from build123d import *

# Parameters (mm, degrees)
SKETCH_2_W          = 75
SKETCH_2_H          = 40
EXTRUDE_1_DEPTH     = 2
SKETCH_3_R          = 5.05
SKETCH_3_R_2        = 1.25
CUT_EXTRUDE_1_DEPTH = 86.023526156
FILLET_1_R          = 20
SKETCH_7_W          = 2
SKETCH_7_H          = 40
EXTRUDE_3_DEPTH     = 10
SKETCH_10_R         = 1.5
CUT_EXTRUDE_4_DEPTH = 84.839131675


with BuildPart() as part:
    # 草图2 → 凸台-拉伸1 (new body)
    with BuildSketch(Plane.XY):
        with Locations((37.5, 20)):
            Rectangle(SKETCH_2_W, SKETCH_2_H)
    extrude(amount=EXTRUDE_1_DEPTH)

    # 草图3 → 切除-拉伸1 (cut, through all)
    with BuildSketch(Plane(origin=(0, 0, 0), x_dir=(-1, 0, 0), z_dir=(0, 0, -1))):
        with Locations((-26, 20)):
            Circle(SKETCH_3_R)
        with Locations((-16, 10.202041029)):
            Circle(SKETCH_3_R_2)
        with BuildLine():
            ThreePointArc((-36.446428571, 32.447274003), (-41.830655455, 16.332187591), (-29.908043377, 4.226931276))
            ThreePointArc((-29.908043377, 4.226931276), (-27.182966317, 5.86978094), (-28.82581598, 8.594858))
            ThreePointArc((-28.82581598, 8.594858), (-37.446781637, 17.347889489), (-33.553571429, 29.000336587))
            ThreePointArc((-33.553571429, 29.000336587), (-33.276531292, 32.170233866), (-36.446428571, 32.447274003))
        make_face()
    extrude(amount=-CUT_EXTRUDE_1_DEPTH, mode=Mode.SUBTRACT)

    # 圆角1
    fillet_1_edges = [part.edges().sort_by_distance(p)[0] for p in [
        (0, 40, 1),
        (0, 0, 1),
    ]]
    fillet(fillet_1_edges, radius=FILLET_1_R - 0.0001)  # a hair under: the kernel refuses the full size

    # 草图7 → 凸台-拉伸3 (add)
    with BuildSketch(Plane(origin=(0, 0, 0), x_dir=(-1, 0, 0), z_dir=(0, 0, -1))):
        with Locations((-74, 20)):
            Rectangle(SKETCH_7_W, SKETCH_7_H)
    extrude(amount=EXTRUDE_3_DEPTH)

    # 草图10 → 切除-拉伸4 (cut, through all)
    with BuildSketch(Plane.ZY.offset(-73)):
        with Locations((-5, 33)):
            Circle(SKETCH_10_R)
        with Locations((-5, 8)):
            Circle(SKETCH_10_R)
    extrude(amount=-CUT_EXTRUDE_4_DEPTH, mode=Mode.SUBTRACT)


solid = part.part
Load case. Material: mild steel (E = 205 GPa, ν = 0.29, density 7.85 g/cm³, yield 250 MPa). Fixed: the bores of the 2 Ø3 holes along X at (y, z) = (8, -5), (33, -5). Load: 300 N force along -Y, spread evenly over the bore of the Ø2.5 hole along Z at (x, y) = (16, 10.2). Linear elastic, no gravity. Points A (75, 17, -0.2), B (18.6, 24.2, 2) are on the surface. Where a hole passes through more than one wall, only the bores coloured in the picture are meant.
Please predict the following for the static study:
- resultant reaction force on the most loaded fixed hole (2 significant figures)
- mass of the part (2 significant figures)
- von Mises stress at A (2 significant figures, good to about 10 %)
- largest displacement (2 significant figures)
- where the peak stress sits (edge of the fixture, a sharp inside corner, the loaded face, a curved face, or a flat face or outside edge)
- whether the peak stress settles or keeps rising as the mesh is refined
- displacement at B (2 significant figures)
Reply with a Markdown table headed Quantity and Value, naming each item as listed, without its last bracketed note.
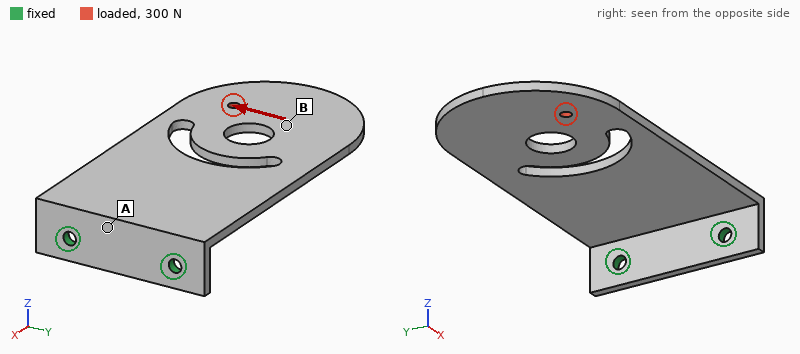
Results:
| Quantity | Value |
|---|---|
| resultant reaction force on the most loaded fixed hole | 670 N |
| mass of the part | 47 g |
| von Mises stress at A | 61 MPa |
| largest displacement | 0.12 mm |
| where the peak stress sits | edge of the fixture |
| whether the peak stress settles or keeps rising as the mesh is refined | keeps rising |
| displacement at B | 0.086 mm |
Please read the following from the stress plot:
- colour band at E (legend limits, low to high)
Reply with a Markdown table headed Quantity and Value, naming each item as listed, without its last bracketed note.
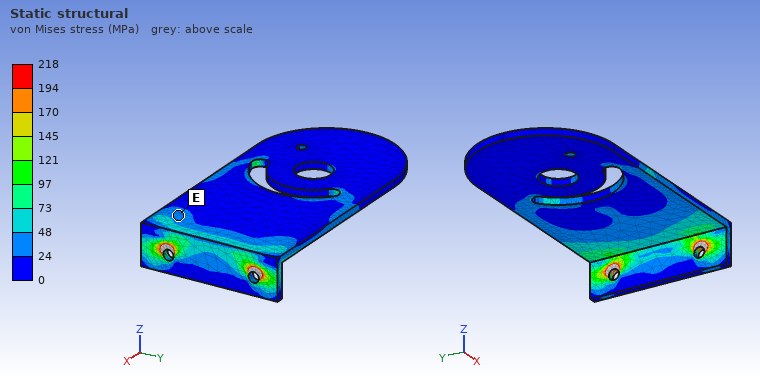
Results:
| Quantity | Value |
|---|---|
| colour band at E | 24 to 48 MPa |
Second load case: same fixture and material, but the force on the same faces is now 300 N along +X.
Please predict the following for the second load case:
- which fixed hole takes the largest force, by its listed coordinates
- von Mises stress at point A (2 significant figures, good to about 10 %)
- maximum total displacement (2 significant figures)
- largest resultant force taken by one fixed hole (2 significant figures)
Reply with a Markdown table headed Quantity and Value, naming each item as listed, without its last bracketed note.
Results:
| Quantity | Value |
|---|---|
| which fixed hole takes the largest force, by its listed coordinates | (8, -5) |
| von Mises stress at point A | 19 MPa |
| maximum total displacement | 87 µm |
| largest resultant force taken by one fixed hole | 270 N |
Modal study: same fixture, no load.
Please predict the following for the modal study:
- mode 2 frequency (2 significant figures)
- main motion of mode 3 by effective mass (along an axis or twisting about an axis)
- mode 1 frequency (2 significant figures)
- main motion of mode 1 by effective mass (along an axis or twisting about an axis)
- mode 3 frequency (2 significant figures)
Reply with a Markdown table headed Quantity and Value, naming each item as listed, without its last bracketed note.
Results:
| Quantity | Value |
|---|---|
| mode 2 frequency | 1200 Hz |
| main motion of mode 3 by effective mass | along Z |
| mode 1 frequency | 290 Hz |
| main motion of mode 1 by effective mass | along Z |
| mode 3 frequency | 1500 Hz |
